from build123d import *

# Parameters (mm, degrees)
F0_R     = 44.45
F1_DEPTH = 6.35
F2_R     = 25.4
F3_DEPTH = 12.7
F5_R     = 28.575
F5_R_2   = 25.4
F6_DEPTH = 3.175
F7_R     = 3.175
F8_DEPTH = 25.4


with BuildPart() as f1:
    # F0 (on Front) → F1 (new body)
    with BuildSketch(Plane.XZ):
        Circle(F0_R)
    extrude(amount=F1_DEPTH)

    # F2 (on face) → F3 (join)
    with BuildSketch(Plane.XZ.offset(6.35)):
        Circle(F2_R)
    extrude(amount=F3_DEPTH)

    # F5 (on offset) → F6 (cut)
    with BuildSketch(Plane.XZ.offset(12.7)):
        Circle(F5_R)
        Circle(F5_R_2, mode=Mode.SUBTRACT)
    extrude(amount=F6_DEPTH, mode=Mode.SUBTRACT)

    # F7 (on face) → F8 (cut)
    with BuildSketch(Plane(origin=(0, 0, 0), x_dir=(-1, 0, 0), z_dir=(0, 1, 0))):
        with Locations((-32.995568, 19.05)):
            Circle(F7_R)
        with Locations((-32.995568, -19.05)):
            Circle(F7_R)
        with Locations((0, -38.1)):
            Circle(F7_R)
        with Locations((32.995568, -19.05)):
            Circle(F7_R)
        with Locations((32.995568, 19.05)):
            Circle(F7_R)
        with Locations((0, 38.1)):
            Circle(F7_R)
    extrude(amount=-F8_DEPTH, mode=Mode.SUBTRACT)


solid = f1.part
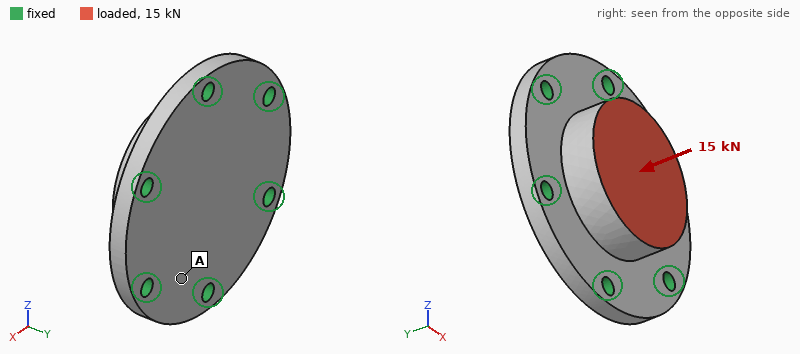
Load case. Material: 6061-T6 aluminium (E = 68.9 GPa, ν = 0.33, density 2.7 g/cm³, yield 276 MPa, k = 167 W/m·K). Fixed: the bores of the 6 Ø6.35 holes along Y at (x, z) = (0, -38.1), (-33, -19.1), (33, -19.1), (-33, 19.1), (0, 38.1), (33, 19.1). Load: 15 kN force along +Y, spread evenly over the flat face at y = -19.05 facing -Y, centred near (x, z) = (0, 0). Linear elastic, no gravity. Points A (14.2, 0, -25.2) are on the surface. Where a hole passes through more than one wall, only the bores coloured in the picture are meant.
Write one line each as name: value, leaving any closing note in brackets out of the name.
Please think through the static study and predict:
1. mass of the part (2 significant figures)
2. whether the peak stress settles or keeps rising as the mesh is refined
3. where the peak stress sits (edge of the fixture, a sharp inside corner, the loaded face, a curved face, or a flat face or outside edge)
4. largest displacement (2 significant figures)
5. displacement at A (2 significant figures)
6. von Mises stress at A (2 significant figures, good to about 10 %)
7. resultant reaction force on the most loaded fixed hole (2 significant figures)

mass of the part: 170 g
whether the peak stress settles or keeps rising as the mesh is refined: keeps rising
where the peak stress sits: edge of the fixture
largest displacement: 38 µm
displacement at A: 24 µm
von Mises stress at A: 29 MPa
resultant reaction force on the most loaded fixed hole: 2.8 kN
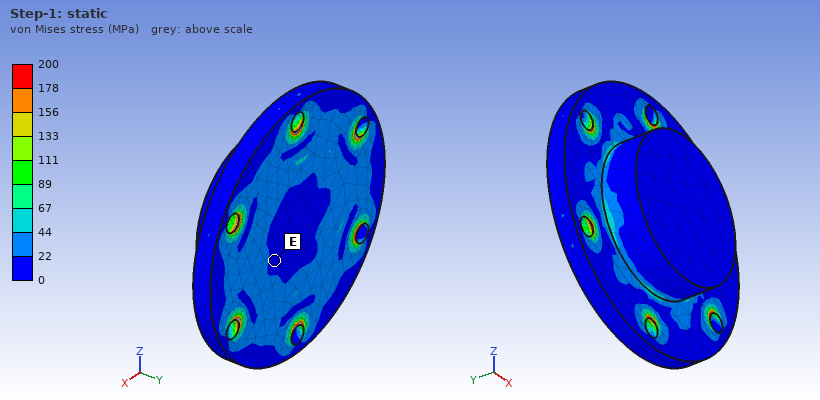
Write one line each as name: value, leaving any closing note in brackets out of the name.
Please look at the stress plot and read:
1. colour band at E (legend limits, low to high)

colour band at E: 0 to 22 MPa
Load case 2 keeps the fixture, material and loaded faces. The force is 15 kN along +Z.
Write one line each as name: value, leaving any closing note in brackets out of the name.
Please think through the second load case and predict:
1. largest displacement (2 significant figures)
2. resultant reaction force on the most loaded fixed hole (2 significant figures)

largest displacement: 35 µm
resultant reaction force on the most loaded fixed hole: 4.3 kN
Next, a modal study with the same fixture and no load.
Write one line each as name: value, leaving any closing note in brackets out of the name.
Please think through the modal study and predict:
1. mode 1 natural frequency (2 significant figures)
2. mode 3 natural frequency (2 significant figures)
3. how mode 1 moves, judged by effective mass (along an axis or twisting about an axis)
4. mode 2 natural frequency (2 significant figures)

mode 1 natural frequency: 9800 Hz
mode 3 natural frequency: 14 kHz
how mode 1 moves, judged by effective mass: along Y
mode 2 natural frequency: 14 kHz
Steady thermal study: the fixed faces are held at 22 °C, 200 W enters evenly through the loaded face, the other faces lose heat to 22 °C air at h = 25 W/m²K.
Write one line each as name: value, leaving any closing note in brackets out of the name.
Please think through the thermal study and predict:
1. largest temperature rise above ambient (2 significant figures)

largest temperature rise above ambient: 30 K
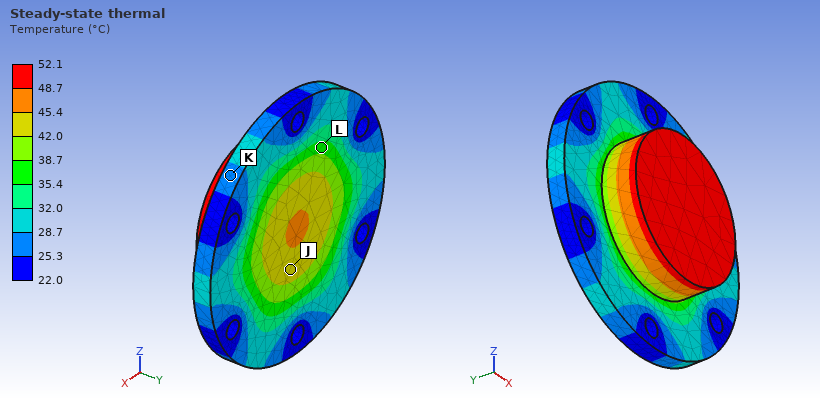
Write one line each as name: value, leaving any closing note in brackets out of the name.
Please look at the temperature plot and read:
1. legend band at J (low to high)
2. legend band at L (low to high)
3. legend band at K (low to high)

legend band at J: 42.0 to 45.4 °C
legend band at L: 35.4 to 38.7 °C
legend band at K: 25.3 to 28.7 °C
